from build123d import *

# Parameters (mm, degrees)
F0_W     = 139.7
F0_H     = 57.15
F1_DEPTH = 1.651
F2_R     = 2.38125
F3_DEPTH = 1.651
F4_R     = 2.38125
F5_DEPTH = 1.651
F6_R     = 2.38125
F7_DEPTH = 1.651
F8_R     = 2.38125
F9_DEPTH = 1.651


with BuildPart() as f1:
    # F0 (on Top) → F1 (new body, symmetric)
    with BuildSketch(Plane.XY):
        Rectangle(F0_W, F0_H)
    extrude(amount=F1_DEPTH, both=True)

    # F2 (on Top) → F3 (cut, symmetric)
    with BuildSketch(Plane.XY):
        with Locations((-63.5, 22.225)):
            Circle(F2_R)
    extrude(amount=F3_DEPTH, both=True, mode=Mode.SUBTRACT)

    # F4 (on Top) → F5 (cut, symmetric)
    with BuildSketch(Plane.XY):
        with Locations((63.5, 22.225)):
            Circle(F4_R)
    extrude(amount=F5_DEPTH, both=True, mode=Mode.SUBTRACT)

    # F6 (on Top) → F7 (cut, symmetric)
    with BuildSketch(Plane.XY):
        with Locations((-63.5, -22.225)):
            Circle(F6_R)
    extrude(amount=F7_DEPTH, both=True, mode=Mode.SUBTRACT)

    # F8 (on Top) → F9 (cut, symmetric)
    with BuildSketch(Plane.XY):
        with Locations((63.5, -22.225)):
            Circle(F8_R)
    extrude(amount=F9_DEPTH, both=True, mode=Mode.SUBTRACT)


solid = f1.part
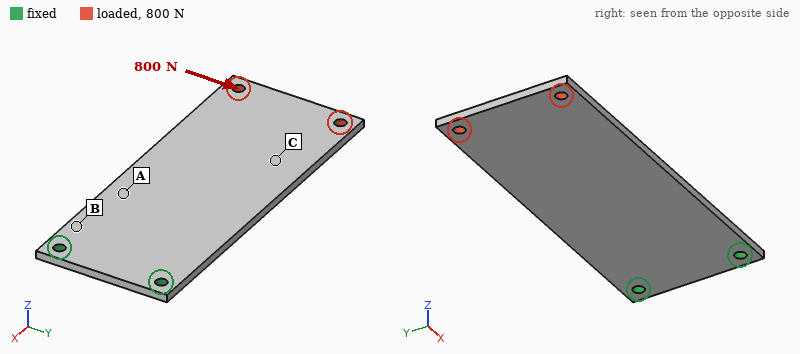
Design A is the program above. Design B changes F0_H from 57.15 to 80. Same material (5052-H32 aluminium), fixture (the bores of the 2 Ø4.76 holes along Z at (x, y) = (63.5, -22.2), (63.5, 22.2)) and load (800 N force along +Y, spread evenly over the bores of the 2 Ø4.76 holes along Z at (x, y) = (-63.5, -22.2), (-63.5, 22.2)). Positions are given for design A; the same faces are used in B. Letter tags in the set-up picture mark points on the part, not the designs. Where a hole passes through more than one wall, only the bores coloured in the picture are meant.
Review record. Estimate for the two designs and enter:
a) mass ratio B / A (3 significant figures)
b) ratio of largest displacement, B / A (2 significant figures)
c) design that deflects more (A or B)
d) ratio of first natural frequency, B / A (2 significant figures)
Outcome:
1.40
0.60
A
1.0
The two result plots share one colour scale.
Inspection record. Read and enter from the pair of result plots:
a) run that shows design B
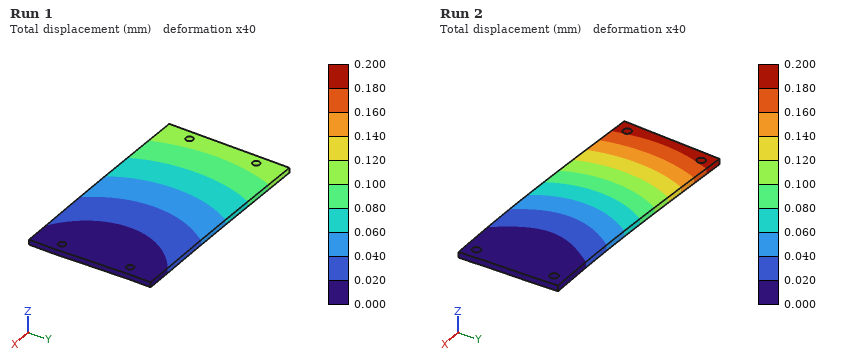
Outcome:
Run 1
